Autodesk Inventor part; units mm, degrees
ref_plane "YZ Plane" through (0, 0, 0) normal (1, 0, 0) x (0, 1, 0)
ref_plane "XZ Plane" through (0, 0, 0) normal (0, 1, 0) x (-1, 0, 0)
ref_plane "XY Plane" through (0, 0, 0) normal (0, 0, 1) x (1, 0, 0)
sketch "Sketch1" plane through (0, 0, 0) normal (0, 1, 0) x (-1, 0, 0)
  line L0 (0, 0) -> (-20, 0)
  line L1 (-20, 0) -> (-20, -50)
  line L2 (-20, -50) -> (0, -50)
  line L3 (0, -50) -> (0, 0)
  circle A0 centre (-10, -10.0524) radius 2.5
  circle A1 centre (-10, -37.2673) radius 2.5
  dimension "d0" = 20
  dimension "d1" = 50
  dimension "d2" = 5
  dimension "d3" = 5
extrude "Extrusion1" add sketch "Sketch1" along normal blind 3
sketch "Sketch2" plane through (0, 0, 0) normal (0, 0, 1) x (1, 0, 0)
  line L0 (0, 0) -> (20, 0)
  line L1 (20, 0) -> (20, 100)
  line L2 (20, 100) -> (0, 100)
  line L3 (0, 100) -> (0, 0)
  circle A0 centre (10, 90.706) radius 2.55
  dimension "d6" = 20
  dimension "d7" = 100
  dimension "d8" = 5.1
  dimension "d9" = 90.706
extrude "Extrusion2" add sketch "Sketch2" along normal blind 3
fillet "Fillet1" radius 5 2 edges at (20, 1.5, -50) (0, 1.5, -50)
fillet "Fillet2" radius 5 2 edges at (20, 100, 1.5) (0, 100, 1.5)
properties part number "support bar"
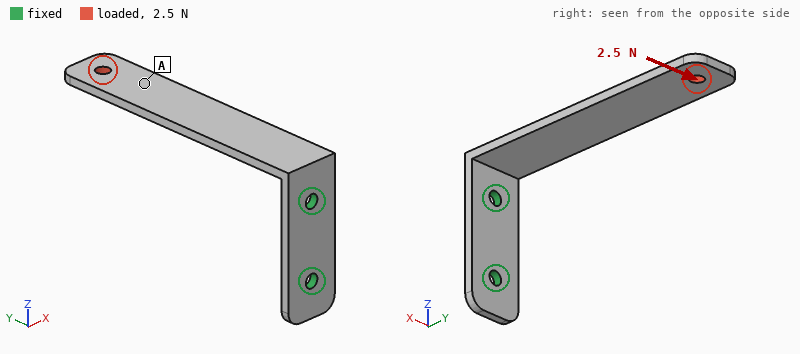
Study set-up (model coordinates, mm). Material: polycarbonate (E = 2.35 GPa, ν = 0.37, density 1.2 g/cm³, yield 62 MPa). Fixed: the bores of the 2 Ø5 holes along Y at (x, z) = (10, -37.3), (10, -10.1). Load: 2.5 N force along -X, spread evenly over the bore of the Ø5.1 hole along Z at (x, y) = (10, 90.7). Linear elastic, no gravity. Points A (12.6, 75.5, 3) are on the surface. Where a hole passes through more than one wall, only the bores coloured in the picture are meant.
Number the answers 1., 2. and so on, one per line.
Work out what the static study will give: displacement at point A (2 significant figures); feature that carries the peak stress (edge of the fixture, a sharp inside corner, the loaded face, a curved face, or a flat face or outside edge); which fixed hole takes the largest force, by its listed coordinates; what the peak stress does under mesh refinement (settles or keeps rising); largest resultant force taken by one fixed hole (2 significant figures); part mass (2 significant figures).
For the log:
1. 0.92 mm
2. edge of the fixture
3. (10, -10.1)
4. keeps rising
5. 3.1 N
6. 11 g
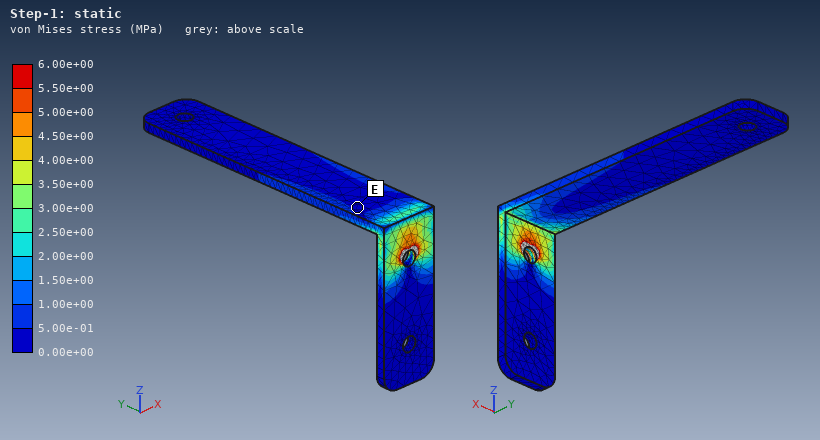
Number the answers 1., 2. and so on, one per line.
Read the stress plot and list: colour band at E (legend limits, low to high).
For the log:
1. 0.00e+00 to 5.00e-01 MPa
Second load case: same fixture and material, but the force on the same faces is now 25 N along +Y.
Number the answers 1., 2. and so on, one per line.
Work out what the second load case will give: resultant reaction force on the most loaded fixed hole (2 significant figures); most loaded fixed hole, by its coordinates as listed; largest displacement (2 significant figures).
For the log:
1. 26 N
2. (10, -10.1)
3. 1.3 mm
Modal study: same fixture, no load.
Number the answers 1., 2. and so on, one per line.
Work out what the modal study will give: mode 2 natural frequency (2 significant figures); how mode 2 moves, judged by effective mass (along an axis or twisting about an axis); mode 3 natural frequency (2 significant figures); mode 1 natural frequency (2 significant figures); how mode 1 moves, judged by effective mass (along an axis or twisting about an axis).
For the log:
1. 140 Hz
2. along X
3. 390 Hz
4. 62 Hz
5. along Z
